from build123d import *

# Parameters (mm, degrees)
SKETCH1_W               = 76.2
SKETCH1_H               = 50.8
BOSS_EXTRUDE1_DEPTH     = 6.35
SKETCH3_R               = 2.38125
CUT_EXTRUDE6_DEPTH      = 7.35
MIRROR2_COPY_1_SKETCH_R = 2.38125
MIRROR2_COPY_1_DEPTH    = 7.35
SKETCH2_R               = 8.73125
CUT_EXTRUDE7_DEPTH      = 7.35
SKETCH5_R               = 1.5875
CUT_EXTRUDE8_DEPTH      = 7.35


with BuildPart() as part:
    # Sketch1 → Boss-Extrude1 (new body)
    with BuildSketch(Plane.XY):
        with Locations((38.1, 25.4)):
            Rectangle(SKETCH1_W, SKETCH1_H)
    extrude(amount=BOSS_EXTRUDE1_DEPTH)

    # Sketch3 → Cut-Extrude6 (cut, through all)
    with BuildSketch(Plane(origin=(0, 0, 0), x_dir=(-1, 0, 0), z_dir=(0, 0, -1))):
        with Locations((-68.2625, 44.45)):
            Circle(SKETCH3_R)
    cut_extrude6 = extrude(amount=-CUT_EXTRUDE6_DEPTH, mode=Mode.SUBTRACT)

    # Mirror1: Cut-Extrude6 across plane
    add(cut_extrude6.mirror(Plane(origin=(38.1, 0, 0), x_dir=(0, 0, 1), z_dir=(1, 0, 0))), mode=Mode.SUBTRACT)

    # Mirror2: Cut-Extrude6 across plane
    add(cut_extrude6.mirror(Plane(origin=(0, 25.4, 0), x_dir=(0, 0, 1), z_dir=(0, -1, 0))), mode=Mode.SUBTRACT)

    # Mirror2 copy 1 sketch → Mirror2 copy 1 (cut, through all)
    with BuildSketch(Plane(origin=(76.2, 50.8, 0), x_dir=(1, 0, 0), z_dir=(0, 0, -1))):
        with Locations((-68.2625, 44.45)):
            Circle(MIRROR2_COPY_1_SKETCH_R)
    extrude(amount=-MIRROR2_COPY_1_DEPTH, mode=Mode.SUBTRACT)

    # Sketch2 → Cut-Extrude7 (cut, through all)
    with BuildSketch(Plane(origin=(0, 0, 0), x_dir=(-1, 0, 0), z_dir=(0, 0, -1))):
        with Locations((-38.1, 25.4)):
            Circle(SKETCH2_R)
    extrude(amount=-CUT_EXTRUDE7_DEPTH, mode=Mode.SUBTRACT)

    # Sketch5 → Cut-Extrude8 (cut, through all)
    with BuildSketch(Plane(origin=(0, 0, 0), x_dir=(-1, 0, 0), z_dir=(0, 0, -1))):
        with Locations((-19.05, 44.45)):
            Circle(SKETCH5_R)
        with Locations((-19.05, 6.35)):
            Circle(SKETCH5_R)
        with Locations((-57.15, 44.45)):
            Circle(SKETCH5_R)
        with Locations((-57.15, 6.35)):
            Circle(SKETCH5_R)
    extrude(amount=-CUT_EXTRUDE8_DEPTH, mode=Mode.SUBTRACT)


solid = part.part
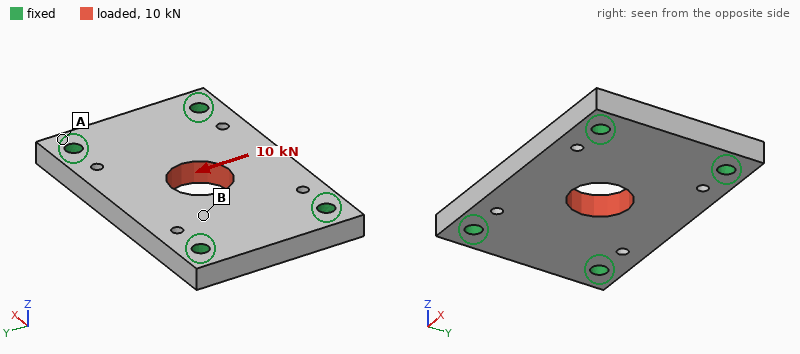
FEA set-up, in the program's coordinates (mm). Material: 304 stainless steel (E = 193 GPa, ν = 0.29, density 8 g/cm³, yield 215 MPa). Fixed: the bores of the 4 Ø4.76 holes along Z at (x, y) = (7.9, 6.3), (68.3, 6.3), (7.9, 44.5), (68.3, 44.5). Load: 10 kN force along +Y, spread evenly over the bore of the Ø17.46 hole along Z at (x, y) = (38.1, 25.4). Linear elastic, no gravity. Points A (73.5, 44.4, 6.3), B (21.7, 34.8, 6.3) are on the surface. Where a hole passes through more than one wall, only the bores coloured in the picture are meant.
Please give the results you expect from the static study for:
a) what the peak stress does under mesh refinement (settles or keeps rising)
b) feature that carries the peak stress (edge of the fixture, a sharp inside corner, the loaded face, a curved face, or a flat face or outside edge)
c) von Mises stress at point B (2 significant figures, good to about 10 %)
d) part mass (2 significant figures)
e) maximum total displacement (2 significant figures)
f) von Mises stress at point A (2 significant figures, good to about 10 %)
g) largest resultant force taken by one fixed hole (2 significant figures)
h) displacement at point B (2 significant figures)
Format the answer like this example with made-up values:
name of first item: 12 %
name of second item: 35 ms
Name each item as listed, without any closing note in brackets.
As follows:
what the peak stress does under mesh refinement: keeps rising
feature that carries the peak stress: edge of the fixture
von Mises stress at point B: 34 MPa
part mass: 180 g
maximum total displacement: 8.2 µm
von Mises stress at point A: 11 MPa
largest resultant force taken by one fixed hole: 3.0 kN
displacement at point B: 4.1 µm
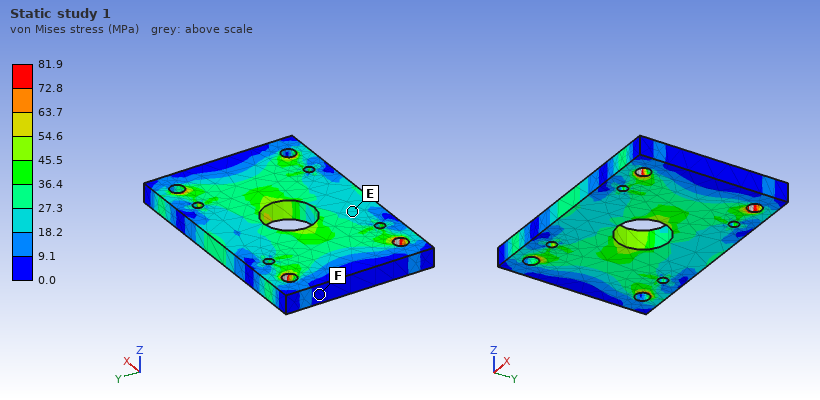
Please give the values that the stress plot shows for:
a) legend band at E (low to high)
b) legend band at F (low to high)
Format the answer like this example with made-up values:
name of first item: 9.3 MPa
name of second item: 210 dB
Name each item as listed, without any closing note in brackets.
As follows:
legend band at E: 18.2 to 27.3 MPa
legend band at F: 0.0 to 9.1 MPa
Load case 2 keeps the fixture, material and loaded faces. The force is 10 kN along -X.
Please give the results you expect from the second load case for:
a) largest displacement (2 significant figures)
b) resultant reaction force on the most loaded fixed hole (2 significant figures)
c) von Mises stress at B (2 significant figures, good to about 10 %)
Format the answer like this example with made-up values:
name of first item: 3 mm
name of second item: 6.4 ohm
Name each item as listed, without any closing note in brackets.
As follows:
largest displacement: 4.2 µm
resultant reaction force on the most loaded fixed hole: 2.6 kN
von Mises stress at B: 24 MPa
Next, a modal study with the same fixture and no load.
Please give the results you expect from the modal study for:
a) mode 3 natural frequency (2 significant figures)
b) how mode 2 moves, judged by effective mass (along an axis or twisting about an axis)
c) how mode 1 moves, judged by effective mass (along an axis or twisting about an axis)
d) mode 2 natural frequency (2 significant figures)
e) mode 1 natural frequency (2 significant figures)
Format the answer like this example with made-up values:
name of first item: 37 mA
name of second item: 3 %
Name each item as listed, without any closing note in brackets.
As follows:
mode 3 natural frequency: 16 kHz
how mode 2 moves, judged by effective mass: twisting about X
how mode 1 moves, judged by effective mass: along Z
mode 2 natural frequency: 10 kHz
mode 1 natural frequency: 7600 Hz
